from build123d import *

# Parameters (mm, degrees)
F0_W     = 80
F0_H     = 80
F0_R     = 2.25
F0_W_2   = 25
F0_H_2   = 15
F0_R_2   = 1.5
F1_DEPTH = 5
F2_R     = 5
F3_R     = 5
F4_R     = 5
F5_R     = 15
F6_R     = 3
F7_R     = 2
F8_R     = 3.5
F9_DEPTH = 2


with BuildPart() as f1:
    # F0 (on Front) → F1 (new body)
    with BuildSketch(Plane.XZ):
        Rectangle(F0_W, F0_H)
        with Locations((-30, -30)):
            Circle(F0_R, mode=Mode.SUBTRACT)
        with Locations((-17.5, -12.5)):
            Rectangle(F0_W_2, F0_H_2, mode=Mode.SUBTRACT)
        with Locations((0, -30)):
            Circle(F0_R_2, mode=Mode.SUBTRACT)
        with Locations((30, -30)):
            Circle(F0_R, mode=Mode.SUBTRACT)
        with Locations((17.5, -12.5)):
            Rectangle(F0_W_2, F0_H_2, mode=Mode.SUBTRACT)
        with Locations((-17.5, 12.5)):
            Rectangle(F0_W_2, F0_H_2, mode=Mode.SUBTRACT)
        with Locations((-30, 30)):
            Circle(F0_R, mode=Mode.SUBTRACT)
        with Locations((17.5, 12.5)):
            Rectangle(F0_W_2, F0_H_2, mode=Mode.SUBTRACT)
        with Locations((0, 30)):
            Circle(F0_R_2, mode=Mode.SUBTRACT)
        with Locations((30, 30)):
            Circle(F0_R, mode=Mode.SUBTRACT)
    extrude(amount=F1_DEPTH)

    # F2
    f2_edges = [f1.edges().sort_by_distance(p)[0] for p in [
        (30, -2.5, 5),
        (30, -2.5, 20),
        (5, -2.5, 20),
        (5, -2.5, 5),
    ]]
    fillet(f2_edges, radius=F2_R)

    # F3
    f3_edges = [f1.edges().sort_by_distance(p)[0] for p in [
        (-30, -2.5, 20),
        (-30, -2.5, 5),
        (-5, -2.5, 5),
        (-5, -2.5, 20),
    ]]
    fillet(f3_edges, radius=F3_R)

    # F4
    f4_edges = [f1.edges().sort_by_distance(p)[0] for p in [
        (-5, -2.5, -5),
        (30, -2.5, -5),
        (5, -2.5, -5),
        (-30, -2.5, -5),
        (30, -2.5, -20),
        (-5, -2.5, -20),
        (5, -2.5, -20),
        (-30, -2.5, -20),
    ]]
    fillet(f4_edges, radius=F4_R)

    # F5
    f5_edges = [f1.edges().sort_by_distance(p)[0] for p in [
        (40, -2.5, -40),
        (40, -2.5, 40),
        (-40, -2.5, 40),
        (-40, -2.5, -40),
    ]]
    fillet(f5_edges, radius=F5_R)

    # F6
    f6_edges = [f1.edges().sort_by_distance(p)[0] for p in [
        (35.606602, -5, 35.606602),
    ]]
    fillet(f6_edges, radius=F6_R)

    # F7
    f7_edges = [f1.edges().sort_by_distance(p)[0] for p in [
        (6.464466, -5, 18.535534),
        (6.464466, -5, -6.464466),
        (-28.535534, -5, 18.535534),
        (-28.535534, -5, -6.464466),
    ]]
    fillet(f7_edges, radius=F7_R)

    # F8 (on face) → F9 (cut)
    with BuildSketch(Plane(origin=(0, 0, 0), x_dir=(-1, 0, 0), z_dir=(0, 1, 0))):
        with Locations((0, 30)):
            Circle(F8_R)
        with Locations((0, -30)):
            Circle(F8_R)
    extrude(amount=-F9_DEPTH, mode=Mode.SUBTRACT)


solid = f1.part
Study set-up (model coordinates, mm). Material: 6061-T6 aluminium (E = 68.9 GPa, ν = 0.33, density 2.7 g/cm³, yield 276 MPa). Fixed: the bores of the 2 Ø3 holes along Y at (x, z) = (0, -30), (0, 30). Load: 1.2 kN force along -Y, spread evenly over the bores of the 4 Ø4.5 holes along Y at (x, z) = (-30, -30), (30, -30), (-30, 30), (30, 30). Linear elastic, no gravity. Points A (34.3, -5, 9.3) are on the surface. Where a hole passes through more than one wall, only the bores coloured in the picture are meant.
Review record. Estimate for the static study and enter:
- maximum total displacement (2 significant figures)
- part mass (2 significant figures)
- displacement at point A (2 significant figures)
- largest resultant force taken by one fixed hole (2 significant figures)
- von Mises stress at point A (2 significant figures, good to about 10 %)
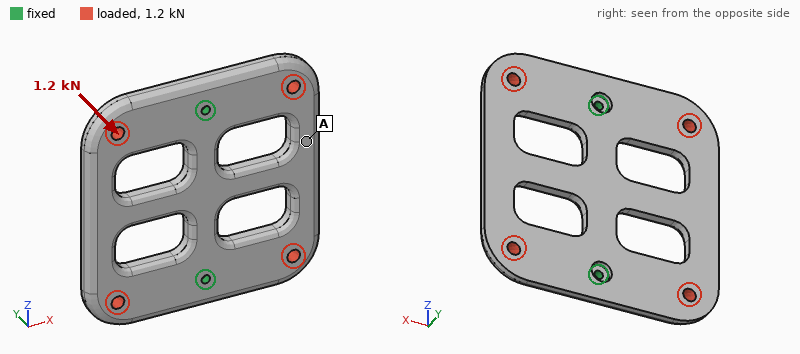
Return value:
0.24 mm
61 g
0.18 mm
600 N
11 MPa
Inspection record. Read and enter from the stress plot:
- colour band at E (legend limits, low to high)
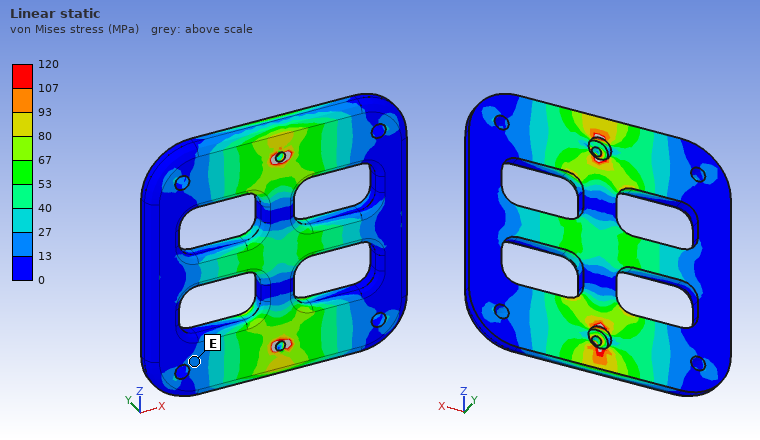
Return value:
13 to 27 MPa
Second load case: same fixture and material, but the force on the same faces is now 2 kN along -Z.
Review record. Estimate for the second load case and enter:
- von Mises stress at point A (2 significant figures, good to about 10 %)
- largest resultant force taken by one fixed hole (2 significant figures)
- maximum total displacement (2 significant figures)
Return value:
6.3 MPa
1.0 kN
18 µm
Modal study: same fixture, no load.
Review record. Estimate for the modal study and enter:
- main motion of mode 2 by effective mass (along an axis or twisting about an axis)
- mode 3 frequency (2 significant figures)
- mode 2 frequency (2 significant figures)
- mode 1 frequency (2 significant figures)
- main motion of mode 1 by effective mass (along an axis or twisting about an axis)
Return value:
along Y
2900 Hz
2100 Hz
1300 Hz
twisting about Z
